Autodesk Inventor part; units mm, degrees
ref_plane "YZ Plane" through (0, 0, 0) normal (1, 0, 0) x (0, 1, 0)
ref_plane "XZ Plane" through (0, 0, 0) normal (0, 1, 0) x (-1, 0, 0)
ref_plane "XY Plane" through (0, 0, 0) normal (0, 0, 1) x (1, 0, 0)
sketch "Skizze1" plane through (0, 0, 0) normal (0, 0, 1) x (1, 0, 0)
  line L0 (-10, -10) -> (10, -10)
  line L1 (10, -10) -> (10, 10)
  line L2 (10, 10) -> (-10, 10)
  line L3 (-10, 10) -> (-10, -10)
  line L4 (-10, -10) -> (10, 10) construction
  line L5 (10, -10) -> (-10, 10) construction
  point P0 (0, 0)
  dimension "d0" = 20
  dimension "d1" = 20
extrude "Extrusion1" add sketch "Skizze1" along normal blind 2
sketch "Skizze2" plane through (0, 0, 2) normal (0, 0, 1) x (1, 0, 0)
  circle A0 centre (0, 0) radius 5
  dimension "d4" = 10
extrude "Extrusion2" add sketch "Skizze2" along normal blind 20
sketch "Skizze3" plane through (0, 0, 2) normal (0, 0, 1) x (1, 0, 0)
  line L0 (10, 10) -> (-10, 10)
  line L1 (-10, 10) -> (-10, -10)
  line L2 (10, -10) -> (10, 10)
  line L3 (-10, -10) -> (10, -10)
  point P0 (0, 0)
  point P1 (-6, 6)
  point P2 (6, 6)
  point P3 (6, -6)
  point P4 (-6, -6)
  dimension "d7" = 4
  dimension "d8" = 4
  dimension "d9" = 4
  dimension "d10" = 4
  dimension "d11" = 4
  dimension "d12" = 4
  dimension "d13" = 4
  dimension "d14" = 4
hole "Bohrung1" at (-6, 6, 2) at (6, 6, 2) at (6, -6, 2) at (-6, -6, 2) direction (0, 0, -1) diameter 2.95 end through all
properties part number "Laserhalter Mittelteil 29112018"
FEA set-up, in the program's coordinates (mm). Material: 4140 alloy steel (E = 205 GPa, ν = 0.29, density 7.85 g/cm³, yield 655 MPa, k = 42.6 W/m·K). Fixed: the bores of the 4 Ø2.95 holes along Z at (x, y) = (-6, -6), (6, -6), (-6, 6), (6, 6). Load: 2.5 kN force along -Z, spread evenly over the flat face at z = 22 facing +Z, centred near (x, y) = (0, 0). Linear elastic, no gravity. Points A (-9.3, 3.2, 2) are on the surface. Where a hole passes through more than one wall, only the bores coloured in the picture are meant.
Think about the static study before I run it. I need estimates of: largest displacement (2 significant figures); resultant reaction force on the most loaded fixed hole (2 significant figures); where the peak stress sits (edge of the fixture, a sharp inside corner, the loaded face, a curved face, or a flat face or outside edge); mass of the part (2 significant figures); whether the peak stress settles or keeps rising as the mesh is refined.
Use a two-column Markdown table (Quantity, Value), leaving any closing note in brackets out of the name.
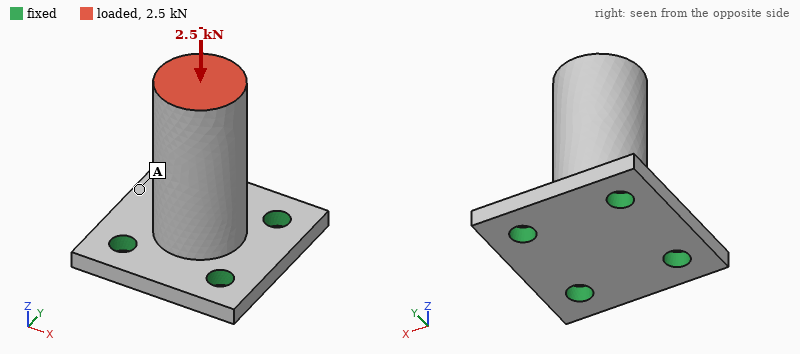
| Quantity | Value |
|---|---|
| largest displacement | 8.0 µm |
| resultant reaction force on the most loaded fixed hole | 660 N |
| where the peak stress sits | edge of the fixture |
| mass of the part | 18 g |
| whether the peak stress settles or keeps rising as the mesh is refined | keeps rising |
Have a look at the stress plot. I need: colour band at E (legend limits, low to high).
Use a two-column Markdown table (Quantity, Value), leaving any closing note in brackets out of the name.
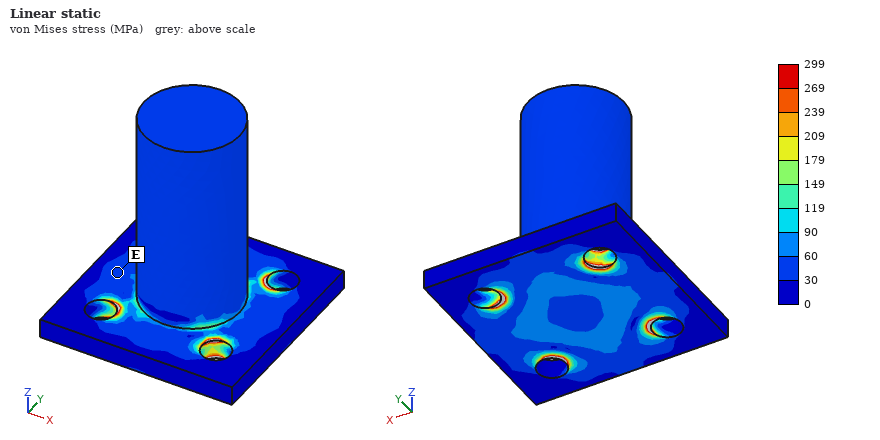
| Quantity | Value |
|---|---|
| colour band at E | 30 to 60 MPa |
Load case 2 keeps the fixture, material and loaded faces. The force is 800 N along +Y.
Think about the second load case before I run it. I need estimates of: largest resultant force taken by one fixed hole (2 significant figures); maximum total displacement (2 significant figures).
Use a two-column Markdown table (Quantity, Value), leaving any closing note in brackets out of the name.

| Quantity | Value |
|---|---|
| largest resultant force taken by one fixed hole | 880 N |
| maximum total displacement | 58 µm |
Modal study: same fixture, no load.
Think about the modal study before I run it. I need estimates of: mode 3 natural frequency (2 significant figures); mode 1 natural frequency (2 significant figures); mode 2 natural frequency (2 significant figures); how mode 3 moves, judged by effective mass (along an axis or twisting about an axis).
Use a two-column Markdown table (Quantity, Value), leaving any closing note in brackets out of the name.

| Quantity | Value |
|---|---|
| mode 3 natural frequency | 28 kHz |
| mode 1 natural frequency | 9600 Hz |
| mode 2 natural frequency | 9600 Hz |
| how mode 3 moves, judged by effective mass | along Z |
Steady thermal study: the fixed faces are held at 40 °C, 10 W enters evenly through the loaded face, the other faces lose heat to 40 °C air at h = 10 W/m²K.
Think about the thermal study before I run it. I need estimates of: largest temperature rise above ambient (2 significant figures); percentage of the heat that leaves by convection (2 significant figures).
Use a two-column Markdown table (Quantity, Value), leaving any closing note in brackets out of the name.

| Quantity | Value |
|---|---|
| largest temperature rise above ambient | 74 K |
| percentage of the heat that leaves by convection | 3.2 % |
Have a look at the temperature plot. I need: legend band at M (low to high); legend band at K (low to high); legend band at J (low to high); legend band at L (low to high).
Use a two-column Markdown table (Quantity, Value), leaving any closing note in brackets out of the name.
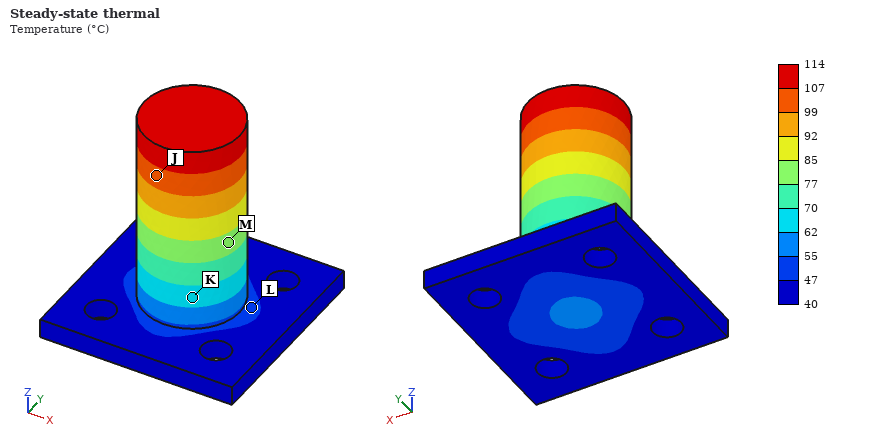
| Quantity | Value |
|---|---|
| legend band at M | 77 to 85 °C |
| legend band at K | 62 to 70 °C |
| legend band at J | 99 to 107 °C |
| legend band at L | 47 to 55 °C |
